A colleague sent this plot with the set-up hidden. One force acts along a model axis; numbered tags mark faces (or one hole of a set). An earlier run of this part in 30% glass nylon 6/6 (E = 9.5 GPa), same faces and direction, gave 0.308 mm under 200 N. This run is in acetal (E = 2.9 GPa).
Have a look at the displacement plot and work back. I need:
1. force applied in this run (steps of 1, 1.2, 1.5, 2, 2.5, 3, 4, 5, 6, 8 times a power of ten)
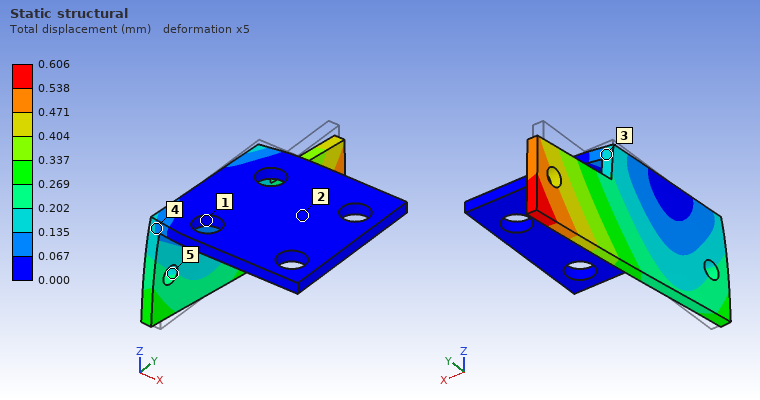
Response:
120 N
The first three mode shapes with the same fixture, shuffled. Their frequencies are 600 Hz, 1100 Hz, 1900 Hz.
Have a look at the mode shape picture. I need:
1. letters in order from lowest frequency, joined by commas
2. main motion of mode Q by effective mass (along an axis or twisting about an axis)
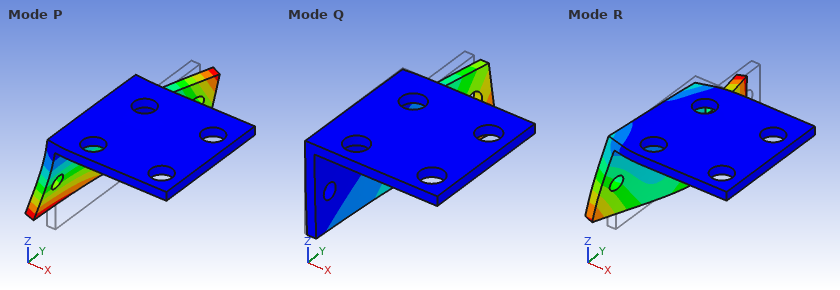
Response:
Q, P, R
along X
